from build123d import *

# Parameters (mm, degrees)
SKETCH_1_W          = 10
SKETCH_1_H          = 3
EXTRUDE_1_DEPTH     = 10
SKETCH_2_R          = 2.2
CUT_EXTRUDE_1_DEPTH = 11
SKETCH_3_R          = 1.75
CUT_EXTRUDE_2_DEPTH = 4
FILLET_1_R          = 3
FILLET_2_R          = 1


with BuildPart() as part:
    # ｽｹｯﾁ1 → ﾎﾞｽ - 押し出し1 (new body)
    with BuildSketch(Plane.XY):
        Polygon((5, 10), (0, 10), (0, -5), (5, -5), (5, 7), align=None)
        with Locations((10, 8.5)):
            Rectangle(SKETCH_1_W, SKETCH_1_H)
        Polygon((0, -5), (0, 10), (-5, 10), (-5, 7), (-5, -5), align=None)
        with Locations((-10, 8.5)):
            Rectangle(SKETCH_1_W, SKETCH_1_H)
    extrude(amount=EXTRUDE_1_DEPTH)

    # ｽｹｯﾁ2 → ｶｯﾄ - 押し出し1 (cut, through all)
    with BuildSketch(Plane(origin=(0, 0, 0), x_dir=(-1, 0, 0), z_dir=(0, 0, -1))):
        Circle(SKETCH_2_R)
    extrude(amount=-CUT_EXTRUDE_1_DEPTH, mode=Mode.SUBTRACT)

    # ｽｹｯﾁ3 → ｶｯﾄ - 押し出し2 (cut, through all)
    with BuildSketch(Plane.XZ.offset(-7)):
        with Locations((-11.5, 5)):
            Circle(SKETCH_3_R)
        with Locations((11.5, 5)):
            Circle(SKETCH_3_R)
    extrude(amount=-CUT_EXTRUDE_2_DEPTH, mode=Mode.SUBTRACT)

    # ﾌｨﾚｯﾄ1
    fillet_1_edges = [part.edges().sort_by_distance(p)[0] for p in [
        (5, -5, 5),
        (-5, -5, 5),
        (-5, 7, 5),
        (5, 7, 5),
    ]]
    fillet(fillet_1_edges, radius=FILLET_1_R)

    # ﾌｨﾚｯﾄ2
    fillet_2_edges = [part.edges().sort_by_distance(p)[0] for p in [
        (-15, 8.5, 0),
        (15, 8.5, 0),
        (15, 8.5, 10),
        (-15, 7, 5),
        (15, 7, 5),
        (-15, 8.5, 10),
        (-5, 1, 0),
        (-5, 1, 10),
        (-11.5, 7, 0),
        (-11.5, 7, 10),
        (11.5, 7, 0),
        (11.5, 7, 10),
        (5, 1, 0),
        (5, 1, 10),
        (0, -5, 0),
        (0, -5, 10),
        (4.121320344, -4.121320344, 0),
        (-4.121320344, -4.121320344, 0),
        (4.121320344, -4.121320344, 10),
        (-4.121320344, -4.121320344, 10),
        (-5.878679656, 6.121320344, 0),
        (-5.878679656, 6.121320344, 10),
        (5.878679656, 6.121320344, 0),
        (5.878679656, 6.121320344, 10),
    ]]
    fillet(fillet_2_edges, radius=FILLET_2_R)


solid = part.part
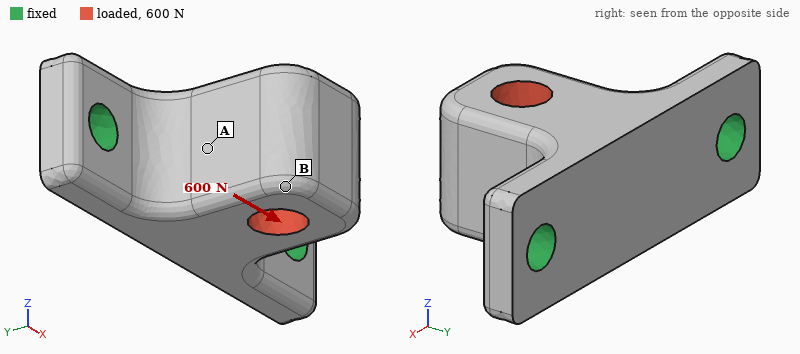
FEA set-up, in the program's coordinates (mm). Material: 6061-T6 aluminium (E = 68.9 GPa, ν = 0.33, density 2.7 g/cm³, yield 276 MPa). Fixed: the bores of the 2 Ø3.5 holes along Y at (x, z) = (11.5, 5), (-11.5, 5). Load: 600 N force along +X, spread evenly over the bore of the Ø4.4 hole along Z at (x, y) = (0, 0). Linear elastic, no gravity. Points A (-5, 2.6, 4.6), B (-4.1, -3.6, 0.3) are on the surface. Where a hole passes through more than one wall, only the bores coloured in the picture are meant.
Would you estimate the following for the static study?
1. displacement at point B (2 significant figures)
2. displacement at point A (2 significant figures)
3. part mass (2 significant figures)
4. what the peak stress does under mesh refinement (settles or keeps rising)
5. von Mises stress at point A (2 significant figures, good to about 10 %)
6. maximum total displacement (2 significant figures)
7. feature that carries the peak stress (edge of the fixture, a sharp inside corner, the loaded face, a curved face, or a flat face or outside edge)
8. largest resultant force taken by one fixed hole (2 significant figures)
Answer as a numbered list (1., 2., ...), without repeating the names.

1. 14 µm
2. 7.2 µm
3. 5.0 g
4. keeps rising
5. 18 MPa
6. 15 µm
7. edge of the fixture
8. 420 N
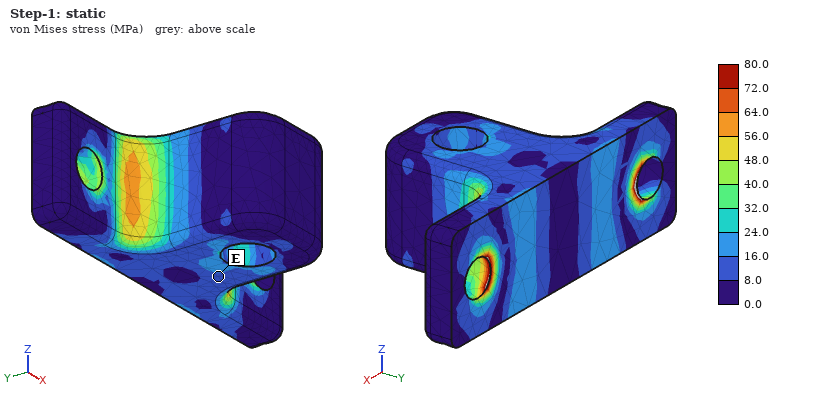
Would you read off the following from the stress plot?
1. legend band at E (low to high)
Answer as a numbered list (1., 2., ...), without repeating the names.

1. 8.0 to 16.0 MPa
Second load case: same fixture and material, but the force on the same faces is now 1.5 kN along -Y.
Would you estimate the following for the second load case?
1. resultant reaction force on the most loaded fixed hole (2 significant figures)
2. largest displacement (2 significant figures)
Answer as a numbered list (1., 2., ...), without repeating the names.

1. 860 N
2. 19 µm
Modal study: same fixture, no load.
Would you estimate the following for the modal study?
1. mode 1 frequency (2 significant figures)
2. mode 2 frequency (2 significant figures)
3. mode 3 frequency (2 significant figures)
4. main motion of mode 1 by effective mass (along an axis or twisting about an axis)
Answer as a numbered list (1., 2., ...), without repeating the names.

1. 10 kHz
2. 24 kHz
3. 25 kHz
4. along Z
